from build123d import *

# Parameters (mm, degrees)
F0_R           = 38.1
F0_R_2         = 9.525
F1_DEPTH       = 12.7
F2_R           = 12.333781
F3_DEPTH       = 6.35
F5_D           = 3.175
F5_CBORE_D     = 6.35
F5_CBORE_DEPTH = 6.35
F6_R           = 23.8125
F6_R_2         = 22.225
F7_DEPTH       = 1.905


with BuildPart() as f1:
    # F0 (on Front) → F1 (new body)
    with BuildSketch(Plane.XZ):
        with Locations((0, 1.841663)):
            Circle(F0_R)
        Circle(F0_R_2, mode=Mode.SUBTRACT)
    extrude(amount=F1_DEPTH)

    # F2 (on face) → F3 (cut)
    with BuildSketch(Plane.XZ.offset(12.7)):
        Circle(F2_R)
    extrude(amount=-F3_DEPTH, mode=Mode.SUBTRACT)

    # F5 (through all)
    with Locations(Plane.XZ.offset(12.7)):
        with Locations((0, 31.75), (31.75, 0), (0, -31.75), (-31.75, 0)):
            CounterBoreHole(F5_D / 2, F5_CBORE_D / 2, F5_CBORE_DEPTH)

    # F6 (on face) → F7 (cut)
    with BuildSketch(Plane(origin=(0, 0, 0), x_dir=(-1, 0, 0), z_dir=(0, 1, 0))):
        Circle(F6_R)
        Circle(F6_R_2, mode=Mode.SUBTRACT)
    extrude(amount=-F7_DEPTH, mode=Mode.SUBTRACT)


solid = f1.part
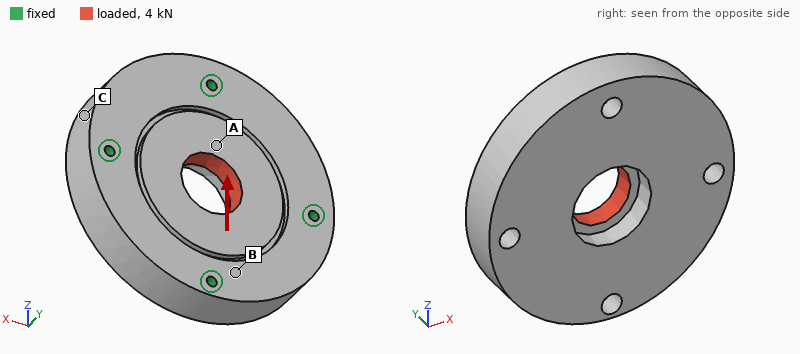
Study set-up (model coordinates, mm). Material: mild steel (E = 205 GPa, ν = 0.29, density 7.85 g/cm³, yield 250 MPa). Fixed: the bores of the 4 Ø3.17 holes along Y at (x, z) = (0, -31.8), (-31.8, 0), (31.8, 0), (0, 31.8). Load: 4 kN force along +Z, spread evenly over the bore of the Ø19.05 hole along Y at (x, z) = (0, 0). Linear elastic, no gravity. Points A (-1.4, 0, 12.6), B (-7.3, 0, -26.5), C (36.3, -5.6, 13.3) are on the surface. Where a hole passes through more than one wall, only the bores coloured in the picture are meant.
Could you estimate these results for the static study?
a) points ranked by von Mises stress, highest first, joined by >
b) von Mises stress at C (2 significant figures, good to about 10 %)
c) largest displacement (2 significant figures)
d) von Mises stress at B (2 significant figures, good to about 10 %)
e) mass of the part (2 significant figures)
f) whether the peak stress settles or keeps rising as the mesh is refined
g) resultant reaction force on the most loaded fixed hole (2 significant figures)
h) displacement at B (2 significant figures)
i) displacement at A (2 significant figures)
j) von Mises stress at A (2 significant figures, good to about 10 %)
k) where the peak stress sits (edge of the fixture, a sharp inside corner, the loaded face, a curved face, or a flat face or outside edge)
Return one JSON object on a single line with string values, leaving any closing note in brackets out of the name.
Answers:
{"points ranked by von Mises stress, highest first, joined by >": "A > B > C", "von Mises stress at C": "2.5 MPa", "largest displacement": "1.4 µm", "von Mises stress at B": "5.5 MPa", "mass of the part": "410 g", "whether the peak stress settles or keeps rising as the mesh is refined": "keeps rising", "resultant reaction force on the most loaded fixed hole": "1.1 kN", "displacement at B": "0.51 µm", "displacement at A": "1.2 µm", "von Mises stress at A": "12 MPa", "where the peak stress sits": "edge of the fixture"}
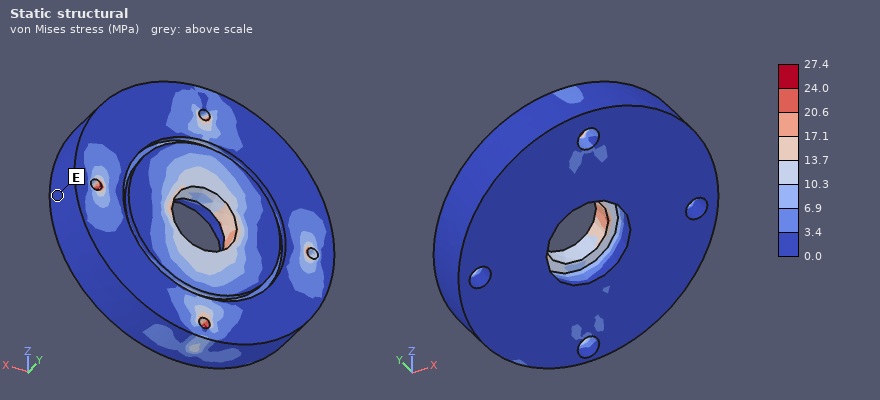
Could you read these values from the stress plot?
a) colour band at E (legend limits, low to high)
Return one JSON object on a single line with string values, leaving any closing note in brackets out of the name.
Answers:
{"colour band at E": "0.0 to 3.4 MPa"}
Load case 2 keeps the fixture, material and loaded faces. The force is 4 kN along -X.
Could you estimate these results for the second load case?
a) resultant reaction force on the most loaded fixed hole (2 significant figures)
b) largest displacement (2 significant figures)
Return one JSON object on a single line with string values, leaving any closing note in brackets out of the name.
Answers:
{"resultant reaction force on the most loaded fixed hole": "1.1 kN", "largest displacement": "1.4 µm"}
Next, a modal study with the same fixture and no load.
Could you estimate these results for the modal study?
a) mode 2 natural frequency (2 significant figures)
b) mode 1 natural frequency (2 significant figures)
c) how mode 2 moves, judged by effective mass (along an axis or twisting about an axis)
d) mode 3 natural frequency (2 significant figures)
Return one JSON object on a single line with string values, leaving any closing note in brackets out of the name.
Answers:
{"mode 2 natural frequency": "14 kHz", "mode 1 natural frequency": "12 kHz", "how mode 2 moves, judged by effective mass": "along Y", "mode 3 natural frequency": "14 kHz"}
